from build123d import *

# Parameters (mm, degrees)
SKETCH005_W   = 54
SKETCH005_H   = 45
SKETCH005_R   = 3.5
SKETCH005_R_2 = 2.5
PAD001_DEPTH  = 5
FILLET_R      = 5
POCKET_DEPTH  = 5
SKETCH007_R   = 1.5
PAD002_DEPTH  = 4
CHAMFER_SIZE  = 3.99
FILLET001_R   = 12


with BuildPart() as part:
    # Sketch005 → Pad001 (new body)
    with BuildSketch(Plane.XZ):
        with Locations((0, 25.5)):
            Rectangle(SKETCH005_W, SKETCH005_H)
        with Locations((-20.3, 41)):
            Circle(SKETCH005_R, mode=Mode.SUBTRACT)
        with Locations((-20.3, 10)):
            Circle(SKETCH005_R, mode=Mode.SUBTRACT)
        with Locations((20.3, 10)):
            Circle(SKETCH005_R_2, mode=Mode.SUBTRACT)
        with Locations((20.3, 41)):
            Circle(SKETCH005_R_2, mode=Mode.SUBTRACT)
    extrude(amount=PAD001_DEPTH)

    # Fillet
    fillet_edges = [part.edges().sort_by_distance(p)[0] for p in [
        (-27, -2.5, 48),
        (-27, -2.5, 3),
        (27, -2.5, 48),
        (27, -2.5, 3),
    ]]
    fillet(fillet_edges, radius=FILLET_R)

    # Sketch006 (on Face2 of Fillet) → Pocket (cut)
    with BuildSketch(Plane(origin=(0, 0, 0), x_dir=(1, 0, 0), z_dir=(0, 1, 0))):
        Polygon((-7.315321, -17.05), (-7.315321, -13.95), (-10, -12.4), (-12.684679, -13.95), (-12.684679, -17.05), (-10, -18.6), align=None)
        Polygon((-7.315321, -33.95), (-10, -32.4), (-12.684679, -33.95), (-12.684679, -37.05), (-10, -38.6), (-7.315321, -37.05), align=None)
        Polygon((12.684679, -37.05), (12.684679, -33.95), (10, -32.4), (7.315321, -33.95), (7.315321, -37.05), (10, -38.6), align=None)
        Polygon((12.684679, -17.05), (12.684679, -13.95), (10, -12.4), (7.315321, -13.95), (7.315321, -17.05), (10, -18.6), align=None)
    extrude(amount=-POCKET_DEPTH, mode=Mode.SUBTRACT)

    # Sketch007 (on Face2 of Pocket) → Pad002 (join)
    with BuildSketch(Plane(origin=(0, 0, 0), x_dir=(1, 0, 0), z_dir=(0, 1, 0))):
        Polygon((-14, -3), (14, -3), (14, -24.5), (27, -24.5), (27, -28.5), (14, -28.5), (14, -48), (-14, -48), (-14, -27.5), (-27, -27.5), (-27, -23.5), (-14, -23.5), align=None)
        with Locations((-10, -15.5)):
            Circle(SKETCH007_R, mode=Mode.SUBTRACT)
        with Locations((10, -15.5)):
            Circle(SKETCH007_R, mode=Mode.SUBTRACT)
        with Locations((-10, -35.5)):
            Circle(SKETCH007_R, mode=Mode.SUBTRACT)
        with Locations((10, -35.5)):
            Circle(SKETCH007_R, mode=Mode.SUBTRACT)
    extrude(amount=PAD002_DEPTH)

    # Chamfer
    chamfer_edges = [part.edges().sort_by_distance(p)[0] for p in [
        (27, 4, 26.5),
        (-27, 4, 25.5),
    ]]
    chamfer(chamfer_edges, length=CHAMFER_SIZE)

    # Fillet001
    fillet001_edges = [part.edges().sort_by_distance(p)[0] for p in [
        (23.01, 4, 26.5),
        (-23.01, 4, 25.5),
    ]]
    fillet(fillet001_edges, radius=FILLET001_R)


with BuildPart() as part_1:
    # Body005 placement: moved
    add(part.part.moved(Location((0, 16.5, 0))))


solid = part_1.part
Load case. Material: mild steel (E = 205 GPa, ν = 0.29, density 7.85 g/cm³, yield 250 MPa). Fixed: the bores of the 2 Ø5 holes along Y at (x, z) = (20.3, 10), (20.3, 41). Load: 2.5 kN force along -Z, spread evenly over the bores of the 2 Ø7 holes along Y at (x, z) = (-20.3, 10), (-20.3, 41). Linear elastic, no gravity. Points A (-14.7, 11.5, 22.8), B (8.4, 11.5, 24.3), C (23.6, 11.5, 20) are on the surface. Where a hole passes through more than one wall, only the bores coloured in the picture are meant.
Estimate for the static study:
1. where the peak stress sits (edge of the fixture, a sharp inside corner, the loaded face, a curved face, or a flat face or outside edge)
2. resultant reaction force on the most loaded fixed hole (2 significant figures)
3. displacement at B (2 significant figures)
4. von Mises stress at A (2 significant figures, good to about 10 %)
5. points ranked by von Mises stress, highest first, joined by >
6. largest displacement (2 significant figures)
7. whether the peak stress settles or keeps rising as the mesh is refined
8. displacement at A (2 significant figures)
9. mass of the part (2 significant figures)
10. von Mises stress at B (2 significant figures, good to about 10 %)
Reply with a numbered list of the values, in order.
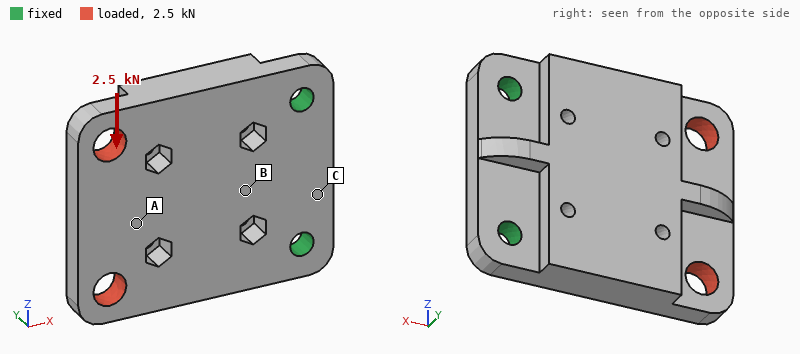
1. edge of the fixture
2. 3.2 kN
3. 3.7 µm
4. 23 MPa
5. B > A > C
6. 21 µm
7. keeps rising
8. 13 µm
9. 130 g
10. 43 MPa
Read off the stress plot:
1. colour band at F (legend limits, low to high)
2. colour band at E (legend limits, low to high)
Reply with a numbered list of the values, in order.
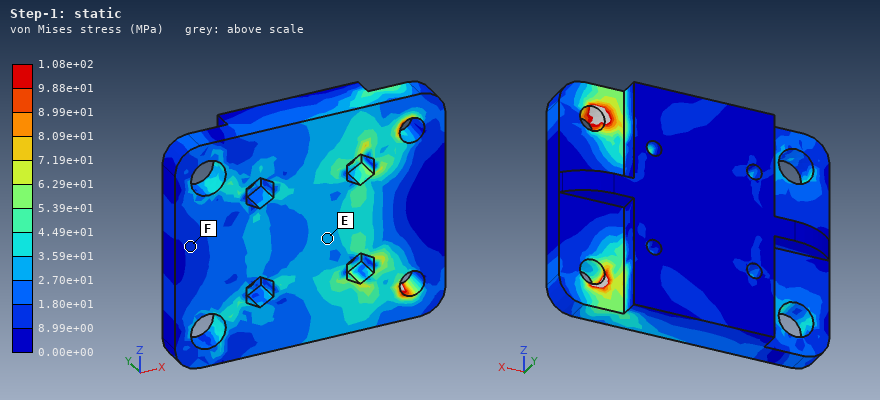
1. 8.99e+00 to 1.80e+01 MPa
2. 2.70e+01 to 3.59e+01 MPa
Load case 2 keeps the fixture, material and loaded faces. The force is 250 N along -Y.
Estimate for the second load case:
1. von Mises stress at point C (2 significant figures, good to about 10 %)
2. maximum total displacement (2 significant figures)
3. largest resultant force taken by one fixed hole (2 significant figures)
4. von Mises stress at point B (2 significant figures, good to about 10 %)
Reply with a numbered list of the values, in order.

1. 16 MPa
2. 43 µm
3. 130 N
4. 16 MPa
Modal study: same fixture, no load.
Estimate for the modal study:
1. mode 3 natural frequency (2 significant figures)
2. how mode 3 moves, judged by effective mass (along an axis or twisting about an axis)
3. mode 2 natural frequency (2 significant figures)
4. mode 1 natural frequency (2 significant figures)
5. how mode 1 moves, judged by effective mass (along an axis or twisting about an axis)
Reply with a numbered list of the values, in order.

1. 10 kHz
2. along Z
3. 6900 Hz
4. 2100 Hz
5. along Y
